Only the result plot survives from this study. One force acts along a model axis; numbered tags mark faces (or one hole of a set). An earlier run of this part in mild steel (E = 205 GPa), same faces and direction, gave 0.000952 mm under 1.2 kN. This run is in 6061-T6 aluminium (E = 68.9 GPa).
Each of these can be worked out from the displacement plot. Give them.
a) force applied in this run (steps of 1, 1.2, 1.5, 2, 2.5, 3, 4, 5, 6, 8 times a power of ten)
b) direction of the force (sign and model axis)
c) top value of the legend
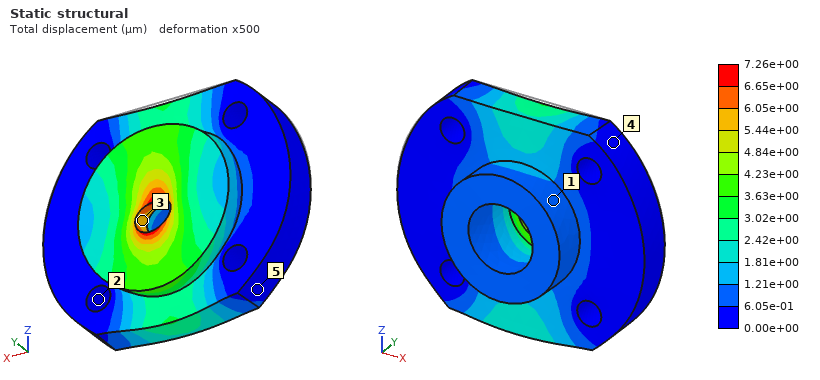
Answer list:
3 kN
-Z
7.26e+00 µm
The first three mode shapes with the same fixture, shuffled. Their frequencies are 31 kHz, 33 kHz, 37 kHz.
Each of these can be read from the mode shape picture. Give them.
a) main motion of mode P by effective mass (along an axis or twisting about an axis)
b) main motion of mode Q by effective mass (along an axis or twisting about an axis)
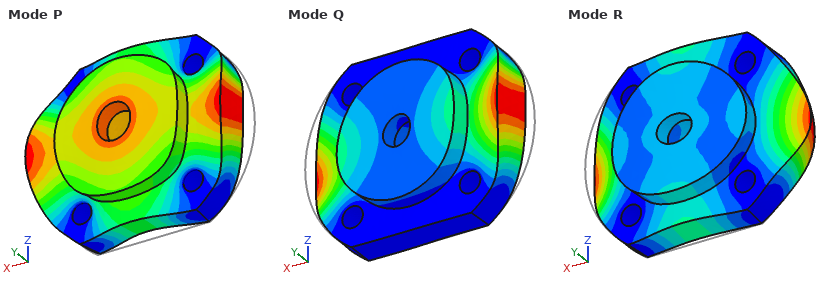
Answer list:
along Y
twisting about Z
